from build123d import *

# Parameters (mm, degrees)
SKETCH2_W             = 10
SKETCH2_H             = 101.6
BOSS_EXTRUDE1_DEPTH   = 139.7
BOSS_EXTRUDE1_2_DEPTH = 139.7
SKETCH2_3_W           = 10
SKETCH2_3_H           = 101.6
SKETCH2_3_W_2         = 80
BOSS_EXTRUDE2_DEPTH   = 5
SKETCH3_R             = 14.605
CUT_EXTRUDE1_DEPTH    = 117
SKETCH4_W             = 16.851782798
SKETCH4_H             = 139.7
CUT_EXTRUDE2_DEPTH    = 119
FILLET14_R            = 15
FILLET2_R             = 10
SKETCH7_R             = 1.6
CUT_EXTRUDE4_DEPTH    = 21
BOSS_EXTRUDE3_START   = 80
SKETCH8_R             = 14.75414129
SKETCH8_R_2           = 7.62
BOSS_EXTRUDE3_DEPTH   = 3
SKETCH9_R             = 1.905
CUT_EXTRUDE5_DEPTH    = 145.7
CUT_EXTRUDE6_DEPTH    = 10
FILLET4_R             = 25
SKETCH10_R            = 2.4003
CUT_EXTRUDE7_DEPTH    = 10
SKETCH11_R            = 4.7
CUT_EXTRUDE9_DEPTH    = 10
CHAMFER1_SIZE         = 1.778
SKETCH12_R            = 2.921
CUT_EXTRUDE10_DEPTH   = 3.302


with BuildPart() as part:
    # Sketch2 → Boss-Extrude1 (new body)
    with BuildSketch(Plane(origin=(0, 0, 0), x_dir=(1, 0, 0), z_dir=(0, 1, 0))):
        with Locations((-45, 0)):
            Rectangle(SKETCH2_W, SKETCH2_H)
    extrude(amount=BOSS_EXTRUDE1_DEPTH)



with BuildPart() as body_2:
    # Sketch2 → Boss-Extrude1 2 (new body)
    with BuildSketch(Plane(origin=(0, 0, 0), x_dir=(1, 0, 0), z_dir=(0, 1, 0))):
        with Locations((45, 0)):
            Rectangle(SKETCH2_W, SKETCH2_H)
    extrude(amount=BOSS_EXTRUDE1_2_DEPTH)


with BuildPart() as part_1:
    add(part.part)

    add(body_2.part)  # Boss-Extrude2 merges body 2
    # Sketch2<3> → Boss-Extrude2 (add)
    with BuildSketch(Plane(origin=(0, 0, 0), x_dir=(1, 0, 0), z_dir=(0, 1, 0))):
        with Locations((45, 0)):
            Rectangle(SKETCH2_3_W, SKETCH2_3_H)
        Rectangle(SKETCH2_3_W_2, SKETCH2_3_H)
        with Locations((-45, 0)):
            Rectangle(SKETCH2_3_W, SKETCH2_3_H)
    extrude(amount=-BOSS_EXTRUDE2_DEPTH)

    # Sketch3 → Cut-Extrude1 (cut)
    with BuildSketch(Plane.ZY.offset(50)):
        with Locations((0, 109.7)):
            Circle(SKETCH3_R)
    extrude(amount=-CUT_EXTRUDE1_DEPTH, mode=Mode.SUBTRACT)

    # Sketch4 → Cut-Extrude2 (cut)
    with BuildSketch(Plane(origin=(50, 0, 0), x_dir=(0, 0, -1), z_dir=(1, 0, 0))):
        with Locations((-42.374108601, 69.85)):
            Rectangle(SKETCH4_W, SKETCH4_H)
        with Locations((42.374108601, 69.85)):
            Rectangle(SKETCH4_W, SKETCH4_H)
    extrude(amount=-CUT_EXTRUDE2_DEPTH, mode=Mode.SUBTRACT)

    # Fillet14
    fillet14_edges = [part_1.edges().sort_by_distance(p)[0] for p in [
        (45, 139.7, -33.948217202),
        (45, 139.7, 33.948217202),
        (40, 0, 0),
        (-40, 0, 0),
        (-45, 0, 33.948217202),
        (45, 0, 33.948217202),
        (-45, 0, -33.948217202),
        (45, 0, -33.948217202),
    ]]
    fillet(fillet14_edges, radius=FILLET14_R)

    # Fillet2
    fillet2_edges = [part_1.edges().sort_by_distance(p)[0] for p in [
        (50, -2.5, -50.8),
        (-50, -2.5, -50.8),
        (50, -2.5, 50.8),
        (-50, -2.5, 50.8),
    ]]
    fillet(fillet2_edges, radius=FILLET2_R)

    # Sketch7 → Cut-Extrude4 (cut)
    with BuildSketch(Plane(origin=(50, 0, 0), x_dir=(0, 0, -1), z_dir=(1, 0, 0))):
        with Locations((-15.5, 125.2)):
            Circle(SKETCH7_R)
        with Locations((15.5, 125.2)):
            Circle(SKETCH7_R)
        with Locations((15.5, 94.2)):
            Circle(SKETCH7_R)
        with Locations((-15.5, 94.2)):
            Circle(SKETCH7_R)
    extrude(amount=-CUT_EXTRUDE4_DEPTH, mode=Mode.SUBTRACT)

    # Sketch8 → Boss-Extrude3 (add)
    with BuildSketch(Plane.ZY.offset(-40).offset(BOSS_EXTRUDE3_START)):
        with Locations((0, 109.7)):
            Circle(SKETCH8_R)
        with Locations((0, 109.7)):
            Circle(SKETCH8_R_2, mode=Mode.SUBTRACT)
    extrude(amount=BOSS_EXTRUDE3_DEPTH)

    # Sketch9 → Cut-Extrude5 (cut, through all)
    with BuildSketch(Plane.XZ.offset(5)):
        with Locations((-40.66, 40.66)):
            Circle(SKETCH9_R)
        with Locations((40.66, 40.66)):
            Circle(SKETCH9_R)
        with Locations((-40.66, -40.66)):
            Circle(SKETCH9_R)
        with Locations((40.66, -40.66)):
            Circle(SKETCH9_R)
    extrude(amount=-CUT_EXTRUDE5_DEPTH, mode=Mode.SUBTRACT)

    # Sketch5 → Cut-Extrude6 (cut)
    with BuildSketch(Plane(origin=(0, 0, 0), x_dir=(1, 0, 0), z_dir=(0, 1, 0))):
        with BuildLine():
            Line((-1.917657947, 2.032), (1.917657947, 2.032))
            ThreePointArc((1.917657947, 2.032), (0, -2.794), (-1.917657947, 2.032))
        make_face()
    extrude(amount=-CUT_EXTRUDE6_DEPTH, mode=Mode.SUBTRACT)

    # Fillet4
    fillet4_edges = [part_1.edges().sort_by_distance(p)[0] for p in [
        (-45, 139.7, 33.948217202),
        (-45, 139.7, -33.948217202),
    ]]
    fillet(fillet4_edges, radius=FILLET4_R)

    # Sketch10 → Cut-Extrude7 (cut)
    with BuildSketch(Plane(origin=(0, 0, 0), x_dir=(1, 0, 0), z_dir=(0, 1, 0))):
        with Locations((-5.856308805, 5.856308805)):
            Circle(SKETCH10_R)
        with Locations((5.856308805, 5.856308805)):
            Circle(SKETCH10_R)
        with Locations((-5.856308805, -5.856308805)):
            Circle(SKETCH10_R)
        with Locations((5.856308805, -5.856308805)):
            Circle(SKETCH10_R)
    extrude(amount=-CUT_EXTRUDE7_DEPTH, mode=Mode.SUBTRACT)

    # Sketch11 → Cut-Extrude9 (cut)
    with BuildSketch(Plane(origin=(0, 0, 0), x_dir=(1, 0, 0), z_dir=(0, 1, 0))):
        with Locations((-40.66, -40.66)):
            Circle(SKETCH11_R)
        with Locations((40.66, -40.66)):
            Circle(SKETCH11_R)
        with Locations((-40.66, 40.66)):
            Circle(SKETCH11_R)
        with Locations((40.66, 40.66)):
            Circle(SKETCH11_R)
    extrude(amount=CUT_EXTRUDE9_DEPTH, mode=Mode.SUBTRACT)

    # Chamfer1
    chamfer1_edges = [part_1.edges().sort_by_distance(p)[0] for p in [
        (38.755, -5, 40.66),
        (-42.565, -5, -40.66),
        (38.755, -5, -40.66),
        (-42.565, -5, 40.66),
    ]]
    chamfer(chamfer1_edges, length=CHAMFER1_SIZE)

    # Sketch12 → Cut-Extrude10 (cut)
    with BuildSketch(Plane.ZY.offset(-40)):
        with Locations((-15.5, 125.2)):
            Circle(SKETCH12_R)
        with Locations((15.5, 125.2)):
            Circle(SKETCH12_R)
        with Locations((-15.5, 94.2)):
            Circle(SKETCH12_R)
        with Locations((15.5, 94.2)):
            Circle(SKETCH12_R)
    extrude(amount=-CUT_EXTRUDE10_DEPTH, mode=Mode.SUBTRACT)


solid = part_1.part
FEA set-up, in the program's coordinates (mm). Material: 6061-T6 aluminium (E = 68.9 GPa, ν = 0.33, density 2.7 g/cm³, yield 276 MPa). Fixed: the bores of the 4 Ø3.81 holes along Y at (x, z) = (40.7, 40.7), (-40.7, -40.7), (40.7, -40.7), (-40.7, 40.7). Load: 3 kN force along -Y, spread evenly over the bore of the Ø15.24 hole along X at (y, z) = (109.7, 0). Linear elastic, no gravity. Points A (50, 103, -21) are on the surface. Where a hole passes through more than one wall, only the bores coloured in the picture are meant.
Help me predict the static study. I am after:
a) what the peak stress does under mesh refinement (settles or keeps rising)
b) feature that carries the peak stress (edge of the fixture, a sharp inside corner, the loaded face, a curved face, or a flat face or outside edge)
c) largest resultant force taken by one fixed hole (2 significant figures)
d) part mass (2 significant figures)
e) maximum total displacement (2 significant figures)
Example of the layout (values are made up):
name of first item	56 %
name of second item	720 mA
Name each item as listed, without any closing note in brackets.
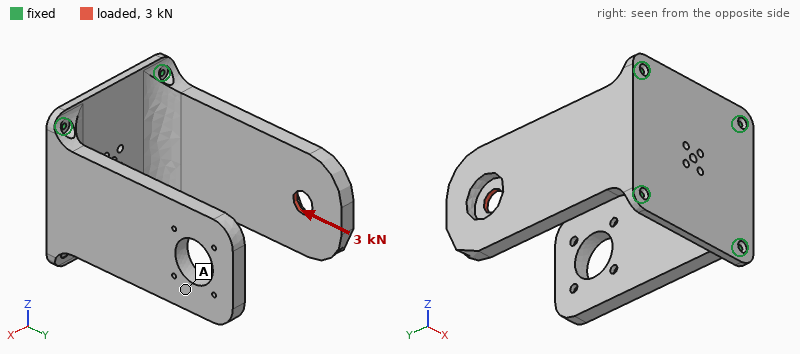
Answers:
what the peak stress does under mesh refinement	keeps rising
feature that carries the peak stress	edge of the fixture
largest resultant force taken by one fixed hole	1.7 kN
part mass	630 g
maximum total displacement	0.18 mm
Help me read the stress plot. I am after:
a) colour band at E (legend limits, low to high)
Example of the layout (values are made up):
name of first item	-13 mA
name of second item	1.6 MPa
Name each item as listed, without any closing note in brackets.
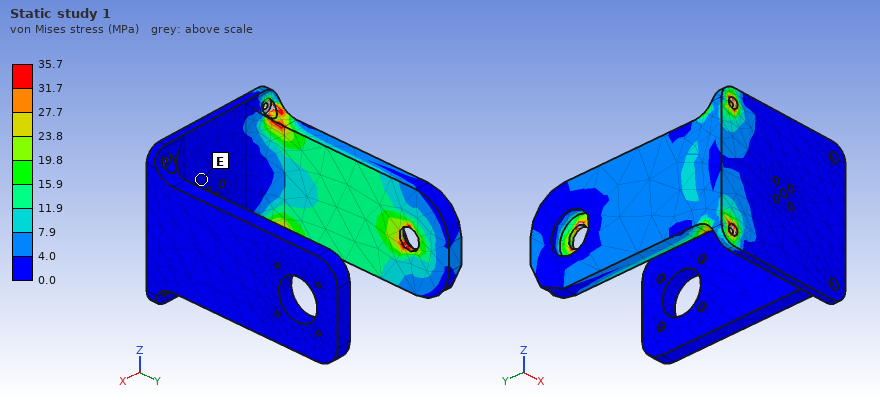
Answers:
colour band at E	0.0 to 4.0 MPa
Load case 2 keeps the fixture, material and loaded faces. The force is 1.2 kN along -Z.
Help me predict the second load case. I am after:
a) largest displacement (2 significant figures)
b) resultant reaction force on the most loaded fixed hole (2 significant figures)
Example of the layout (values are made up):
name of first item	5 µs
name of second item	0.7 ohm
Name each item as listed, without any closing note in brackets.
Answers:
largest displacement	0.11 mm
resultant reaction force on the most loaded fixed hole	1.8 kN
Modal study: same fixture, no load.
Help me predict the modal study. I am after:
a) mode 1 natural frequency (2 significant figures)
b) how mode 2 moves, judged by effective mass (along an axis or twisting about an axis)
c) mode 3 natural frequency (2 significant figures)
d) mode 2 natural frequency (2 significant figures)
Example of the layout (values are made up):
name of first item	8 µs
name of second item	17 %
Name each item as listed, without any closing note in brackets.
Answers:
mode 1 natural frequency	300 Hz
how mode 2 moves, judged by effective mass	along X
mode 3 natural frequency	1700 Hz
mode 2 natural frequency	360 Hz
